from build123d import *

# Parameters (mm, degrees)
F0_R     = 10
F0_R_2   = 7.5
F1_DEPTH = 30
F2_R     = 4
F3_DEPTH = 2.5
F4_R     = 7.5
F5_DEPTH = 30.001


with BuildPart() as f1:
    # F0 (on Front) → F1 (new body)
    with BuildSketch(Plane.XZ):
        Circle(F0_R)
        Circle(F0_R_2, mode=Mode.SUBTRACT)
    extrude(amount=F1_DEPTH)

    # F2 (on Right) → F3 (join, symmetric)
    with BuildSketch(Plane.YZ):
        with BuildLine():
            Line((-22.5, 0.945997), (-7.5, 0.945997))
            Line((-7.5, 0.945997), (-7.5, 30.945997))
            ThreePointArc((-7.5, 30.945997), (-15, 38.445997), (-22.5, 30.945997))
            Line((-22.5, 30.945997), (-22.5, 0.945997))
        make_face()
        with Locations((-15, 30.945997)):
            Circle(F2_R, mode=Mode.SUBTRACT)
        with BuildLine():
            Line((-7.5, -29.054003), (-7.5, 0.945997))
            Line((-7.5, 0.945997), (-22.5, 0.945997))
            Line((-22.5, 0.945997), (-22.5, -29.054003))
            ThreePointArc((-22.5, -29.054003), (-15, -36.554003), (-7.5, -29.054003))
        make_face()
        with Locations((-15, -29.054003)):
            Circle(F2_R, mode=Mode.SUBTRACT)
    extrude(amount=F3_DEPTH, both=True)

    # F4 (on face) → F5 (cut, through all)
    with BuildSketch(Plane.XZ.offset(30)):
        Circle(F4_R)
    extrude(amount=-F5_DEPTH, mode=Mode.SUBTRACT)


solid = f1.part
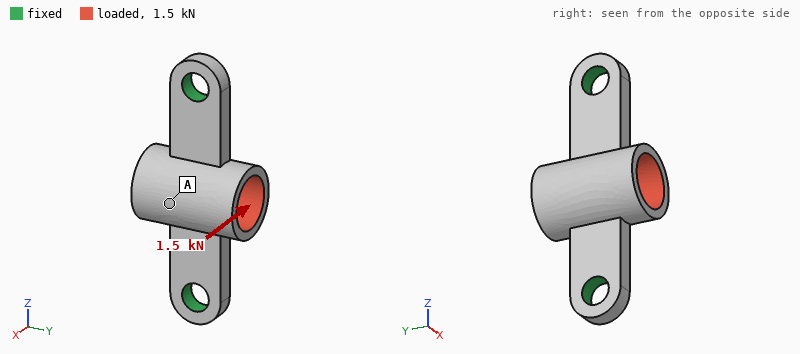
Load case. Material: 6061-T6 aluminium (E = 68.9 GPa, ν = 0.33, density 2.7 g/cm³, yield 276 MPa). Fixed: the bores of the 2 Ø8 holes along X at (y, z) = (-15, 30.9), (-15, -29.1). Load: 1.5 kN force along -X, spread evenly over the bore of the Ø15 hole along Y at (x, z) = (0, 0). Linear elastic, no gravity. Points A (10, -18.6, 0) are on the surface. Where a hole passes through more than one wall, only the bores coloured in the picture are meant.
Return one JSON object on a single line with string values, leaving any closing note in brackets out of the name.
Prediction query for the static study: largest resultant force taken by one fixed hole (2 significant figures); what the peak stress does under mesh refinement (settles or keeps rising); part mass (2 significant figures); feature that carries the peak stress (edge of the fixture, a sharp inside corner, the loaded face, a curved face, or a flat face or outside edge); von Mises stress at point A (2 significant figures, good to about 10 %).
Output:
{"largest resultant force taken by one fixed hole": "780 N", "what the peak stress does under mesh refinement": "keeps rising", "part mass": "20 g", "feature that carries the peak stress": "edge of the fixture", "von Mises stress at point A": "16 MPa"}
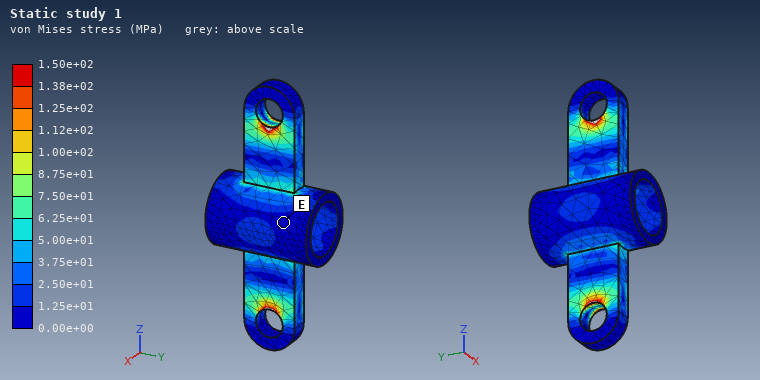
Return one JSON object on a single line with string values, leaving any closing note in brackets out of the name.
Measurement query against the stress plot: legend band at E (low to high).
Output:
{"legend band at E": "0.00e+00 to 1.25e+01 MPa"}
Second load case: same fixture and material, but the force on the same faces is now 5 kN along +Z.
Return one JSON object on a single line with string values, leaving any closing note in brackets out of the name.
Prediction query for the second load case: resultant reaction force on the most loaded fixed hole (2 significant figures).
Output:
{"resultant reaction force on the most loaded fixed hole": "2.5 kN"}
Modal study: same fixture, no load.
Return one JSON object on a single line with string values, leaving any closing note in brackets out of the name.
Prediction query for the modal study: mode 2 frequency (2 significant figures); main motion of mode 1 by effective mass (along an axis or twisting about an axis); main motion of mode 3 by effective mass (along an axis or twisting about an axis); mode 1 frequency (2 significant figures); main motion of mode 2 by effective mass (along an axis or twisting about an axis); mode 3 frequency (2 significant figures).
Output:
{"mode 2 frequency": "7000 Hz", "main motion of mode 1 by effective mass": "twisting about Z", "main motion of mode 3 by effective mass": "along Y", "mode 1 frequency": "5700 Hz", "main motion of mode 2 by effective mass": "along X", "mode 3 frequency": "10 kHz"}
